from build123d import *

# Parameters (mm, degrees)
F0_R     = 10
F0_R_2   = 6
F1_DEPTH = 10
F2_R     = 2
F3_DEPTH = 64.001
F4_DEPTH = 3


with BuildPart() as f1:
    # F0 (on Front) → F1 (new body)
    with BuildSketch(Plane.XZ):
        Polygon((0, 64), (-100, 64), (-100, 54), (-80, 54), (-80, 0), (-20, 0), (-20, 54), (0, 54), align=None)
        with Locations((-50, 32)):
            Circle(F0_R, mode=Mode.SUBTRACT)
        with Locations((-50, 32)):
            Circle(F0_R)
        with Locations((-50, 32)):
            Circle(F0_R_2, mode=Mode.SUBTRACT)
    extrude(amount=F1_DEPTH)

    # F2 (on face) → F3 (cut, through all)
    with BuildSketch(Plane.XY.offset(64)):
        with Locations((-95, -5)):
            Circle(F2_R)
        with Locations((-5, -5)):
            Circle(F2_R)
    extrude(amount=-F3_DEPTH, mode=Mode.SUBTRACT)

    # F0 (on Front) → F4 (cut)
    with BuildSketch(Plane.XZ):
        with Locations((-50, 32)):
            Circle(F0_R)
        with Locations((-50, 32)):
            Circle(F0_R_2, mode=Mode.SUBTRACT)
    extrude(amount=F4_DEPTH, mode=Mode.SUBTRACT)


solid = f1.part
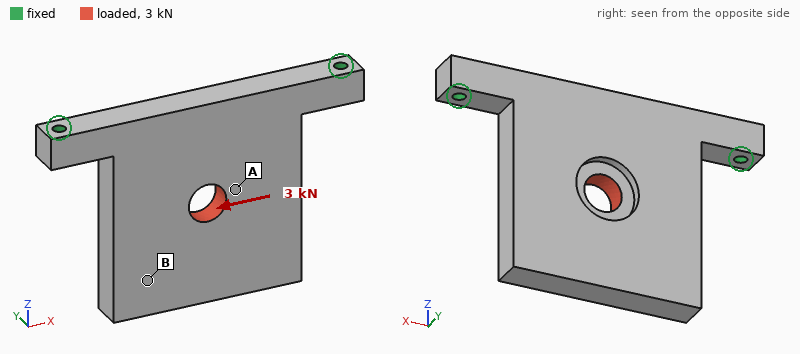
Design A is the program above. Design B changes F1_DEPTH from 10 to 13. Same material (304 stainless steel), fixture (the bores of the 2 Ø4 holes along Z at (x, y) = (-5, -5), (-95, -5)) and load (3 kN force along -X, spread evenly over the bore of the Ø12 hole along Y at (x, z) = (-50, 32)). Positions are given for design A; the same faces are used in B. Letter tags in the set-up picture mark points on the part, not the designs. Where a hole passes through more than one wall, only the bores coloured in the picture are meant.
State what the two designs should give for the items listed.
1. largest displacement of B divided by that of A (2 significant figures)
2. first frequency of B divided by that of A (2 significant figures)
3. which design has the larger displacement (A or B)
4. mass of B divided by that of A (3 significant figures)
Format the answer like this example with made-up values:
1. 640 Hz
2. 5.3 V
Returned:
1. 0.79
2. 1.1
3. A
4. 1.31
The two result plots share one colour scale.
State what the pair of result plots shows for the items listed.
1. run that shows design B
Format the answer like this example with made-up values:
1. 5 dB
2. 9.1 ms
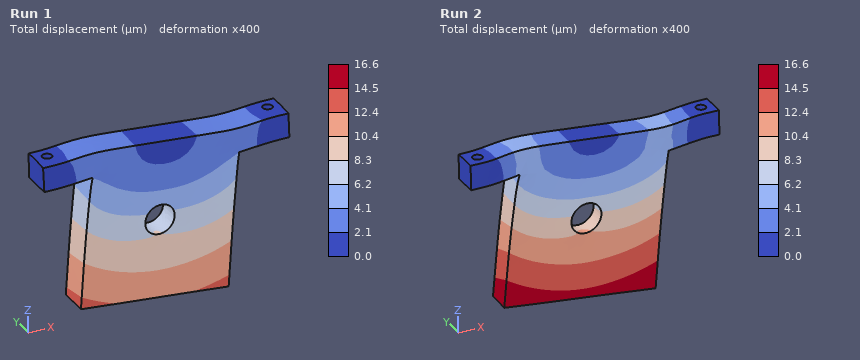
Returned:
1. Run 1
